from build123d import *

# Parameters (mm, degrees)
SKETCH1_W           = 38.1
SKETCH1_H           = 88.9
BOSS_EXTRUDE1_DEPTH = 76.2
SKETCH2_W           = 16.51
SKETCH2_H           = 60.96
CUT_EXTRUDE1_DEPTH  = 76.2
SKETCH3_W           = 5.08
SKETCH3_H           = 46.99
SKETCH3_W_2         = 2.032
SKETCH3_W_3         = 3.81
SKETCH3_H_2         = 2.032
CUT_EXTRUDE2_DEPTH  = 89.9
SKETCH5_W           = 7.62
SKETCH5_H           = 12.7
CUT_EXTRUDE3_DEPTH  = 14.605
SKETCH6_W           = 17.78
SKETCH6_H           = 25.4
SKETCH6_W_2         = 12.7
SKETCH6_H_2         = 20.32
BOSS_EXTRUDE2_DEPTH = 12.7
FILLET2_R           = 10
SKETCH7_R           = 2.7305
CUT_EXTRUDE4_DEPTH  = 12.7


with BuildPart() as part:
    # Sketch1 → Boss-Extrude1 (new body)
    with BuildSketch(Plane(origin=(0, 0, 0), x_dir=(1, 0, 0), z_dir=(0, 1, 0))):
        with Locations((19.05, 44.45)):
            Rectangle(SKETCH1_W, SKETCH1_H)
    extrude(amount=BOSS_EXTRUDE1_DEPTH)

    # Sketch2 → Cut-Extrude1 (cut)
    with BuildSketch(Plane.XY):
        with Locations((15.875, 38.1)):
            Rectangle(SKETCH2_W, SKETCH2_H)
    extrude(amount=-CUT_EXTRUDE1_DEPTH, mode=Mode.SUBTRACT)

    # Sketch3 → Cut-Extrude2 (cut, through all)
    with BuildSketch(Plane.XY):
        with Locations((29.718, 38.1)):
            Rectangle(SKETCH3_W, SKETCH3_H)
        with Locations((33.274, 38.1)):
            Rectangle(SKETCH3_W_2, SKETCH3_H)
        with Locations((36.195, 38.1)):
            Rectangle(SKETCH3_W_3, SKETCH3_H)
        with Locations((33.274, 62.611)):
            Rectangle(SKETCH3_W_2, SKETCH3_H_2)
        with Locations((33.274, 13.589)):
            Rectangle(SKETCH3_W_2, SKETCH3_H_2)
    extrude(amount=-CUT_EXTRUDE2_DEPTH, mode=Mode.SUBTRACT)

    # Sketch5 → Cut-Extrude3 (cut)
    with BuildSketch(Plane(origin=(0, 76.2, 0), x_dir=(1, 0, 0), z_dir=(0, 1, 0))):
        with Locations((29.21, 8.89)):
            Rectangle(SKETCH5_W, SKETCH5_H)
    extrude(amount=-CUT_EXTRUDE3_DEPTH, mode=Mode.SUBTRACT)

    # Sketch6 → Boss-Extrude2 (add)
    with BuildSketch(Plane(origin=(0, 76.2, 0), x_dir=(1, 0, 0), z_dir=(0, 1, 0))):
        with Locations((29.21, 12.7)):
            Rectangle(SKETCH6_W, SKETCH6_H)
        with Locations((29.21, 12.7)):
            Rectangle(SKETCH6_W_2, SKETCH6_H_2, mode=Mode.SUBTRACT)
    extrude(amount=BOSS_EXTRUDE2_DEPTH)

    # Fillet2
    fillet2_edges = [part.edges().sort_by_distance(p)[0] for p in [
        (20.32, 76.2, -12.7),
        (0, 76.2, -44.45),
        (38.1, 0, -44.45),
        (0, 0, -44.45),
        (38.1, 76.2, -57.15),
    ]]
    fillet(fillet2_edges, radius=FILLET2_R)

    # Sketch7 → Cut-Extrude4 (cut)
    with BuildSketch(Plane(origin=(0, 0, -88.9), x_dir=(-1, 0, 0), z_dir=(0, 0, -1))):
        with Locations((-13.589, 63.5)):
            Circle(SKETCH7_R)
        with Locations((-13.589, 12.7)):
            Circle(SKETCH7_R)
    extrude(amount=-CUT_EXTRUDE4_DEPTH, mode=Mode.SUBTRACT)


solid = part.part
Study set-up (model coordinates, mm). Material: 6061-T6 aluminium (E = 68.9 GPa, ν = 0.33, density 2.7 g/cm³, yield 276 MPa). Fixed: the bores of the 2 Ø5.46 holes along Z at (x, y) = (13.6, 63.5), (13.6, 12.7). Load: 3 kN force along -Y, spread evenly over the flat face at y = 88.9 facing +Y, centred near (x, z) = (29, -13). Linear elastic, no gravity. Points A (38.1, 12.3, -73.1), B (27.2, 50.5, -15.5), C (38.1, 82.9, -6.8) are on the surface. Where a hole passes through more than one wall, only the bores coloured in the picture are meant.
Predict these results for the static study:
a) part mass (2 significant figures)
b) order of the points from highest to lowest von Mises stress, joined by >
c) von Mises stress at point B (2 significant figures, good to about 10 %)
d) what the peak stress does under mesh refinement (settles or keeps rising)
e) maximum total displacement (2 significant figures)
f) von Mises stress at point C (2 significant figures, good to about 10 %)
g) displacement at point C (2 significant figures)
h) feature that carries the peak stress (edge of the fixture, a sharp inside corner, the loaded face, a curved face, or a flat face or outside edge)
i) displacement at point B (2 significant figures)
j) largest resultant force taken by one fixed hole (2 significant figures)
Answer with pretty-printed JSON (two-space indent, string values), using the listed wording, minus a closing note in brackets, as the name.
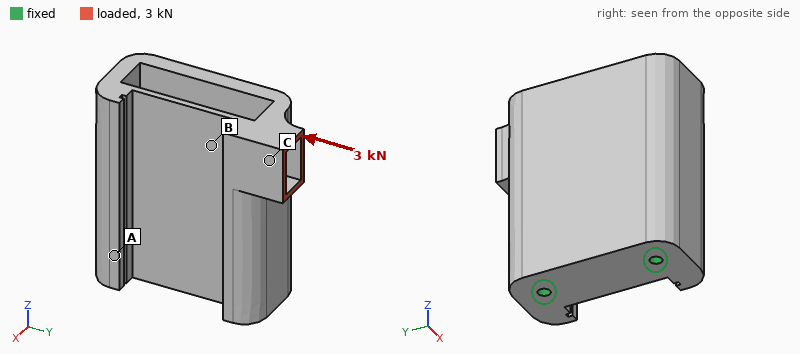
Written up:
{
  "part mass": "350 g",
  "order of the points from highest to lowest von Mises stress, joined by >": "B > C > A",
  "von Mises stress at point B": "29 MPa",
  "what the peak stress does under mesh refinement": "keeps rising",
  "maximum total displacement": "0.11 mm",
  "von Mises stress at point C": "16 MPa",
  "displacement at point C": "0.095 mm",
  "feature that carries the peak stress": "a sharp inside corner",
  "displacement at point B": "0.048 mm",
  "largest resultant force taken by one fixed hole": "4.0 kN"
}
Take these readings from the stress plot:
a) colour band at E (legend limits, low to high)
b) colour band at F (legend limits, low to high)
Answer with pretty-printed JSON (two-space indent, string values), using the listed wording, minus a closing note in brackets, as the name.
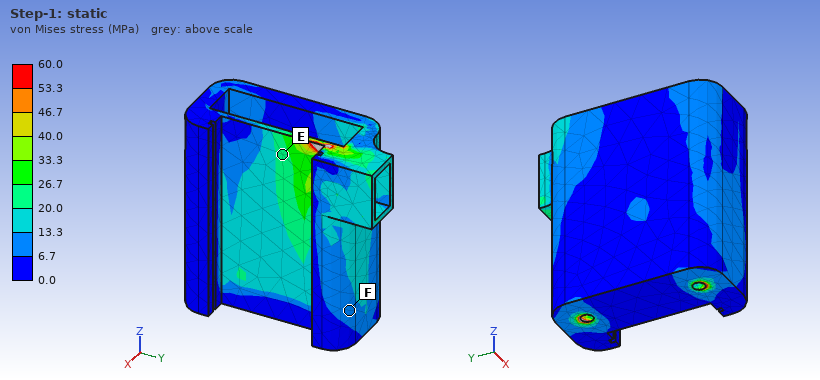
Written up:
{
  "colour band at E": "20.0 to 26.7 MPa",
  "colour band at F": "6.7 to 13.3 MPa"
}
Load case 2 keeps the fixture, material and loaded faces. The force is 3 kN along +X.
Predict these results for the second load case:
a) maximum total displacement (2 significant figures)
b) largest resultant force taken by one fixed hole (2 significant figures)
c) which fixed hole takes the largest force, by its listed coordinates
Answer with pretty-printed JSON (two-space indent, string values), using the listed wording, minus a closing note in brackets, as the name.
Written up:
{
  "maximum total displacement": "0.39 mm",
  "largest resultant force taken by one fixed hole": "4.2 kN",
  "which fixed hole takes the largest force, by its listed coordinates": "(13.6, 63.5)"
}
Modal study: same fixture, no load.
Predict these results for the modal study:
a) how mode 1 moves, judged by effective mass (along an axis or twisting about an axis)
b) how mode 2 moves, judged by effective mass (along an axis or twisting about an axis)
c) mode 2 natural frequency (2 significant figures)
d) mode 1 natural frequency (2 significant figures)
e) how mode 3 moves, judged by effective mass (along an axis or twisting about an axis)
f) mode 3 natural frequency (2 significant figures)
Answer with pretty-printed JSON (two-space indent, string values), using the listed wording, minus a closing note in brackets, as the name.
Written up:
{
  "how mode 1 moves, judged by effective mass": "along X",
  "how mode 2 moves, judged by effective mass": "twisting about Z",
  "mode 2 natural frequency": "3300 Hz",
  "mode 1 natural frequency": "1700 Hz",
  "how mode 3 moves, judged by effective mass": "along Y",
  "mode 3 natural frequency": "4000 Hz"
}
